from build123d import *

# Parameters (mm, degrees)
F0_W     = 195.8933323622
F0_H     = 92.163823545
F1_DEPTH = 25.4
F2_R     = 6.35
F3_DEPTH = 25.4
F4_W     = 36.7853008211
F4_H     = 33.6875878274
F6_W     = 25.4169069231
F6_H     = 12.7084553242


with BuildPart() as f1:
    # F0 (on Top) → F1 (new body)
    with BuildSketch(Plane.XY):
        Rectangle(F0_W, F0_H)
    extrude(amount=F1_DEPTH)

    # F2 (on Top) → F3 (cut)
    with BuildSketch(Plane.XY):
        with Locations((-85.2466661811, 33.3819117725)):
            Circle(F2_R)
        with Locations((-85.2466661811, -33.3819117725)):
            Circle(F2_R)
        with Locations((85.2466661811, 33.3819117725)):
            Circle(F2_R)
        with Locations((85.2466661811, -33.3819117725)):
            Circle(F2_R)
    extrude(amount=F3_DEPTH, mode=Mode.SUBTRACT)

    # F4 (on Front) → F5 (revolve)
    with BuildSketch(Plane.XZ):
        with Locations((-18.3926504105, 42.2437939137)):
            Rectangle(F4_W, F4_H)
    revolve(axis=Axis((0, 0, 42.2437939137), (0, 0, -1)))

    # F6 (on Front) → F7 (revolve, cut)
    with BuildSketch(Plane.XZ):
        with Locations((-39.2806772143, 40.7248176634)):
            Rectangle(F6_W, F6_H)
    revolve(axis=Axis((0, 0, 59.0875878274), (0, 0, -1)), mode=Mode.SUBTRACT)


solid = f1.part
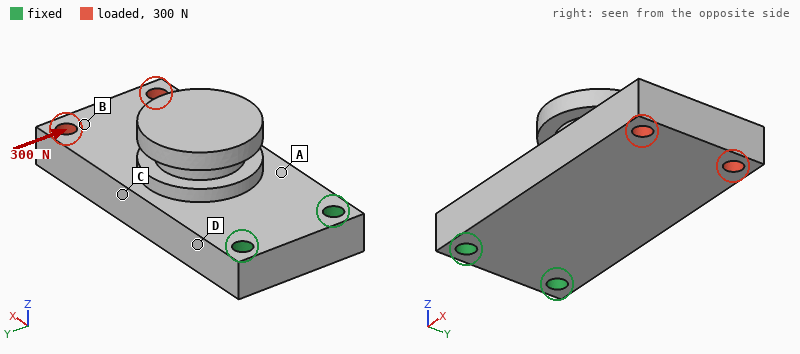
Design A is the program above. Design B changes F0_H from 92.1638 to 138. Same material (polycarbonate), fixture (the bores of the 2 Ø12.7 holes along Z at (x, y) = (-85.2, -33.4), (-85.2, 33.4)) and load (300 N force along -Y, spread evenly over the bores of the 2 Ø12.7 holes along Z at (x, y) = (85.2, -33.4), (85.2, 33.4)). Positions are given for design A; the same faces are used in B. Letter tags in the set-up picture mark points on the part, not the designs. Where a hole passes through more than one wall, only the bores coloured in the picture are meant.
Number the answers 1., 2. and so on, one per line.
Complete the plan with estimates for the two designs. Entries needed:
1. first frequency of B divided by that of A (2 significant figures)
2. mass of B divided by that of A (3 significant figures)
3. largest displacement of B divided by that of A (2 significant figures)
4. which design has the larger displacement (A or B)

1. 0.98
2. 1.41
3. 0.61
4. A
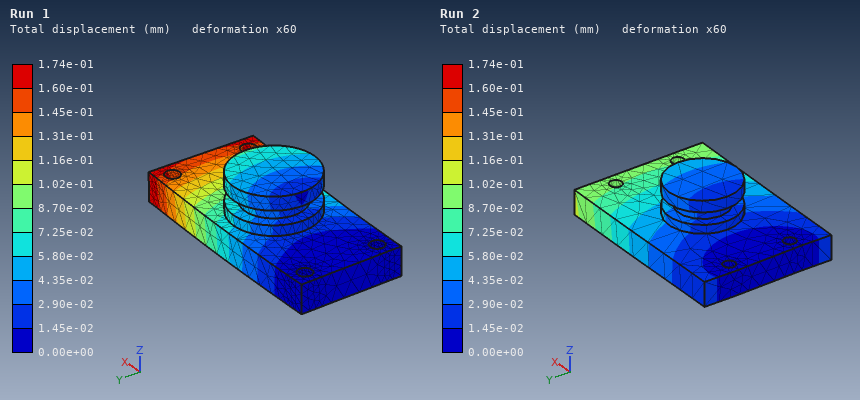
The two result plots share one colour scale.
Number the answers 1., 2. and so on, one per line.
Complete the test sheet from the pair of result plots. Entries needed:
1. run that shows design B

1. Run 2
